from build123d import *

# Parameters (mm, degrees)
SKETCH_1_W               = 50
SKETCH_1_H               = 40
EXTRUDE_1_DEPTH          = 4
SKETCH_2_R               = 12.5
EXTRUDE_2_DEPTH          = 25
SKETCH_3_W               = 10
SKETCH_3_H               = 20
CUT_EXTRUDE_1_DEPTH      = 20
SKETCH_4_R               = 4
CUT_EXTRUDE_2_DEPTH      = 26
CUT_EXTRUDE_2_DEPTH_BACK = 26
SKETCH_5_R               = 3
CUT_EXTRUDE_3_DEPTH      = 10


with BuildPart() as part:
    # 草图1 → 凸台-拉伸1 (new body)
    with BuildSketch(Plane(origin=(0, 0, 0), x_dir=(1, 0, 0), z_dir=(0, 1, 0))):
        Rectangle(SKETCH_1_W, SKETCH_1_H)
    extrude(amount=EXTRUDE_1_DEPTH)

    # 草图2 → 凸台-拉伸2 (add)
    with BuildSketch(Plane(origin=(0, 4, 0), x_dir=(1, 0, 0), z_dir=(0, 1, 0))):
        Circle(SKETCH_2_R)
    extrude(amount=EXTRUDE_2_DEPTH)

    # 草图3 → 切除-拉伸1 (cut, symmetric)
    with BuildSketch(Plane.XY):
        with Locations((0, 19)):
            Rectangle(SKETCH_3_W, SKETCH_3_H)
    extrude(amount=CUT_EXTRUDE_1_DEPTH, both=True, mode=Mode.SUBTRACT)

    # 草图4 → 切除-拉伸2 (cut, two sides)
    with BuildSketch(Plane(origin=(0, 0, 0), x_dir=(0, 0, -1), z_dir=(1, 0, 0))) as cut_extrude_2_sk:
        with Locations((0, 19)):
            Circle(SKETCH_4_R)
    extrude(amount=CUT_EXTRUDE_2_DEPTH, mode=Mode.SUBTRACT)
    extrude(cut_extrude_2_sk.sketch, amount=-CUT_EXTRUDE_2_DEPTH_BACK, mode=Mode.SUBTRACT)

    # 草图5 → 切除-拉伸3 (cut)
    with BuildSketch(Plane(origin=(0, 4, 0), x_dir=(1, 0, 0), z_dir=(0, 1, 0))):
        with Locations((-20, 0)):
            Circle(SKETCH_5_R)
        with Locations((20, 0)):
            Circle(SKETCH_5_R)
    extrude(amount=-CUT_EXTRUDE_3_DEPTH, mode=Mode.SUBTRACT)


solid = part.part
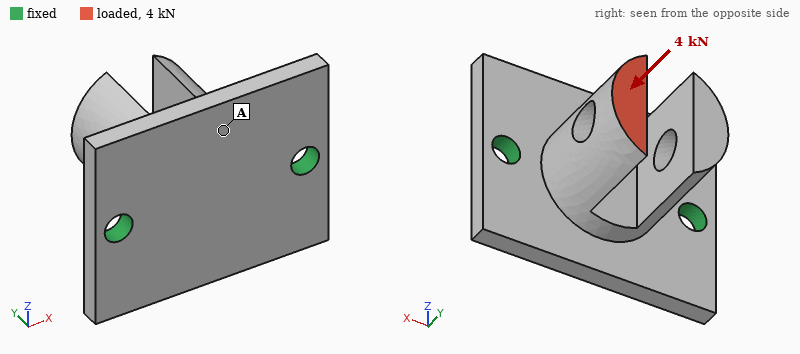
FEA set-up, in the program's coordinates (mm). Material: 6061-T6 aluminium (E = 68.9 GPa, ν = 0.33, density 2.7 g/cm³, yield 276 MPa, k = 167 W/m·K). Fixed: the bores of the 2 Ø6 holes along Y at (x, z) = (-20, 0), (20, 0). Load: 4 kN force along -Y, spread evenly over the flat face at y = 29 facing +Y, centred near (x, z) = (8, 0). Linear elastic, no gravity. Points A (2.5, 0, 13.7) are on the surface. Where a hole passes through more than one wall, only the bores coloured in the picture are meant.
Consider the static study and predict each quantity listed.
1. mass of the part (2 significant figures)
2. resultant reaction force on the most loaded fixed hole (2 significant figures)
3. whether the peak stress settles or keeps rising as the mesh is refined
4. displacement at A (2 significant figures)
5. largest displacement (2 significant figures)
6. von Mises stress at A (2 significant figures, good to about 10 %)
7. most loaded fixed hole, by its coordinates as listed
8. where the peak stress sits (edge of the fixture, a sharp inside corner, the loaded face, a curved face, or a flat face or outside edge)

39 g
3.2 kN
keeps rising
38 µm
64 µm
28 MPa
(20, 0)
edge of the fixture
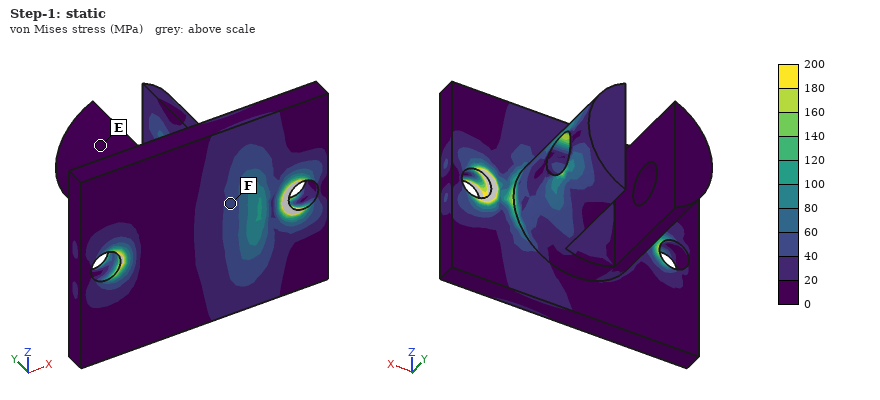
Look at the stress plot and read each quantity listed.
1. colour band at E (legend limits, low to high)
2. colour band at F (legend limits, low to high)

0 to 20 MPa
40 to 60 MPa
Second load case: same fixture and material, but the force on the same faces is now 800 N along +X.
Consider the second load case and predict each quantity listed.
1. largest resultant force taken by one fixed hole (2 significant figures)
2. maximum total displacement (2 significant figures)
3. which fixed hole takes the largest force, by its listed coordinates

1.1 kN
0.18 mm
(-20, 0)
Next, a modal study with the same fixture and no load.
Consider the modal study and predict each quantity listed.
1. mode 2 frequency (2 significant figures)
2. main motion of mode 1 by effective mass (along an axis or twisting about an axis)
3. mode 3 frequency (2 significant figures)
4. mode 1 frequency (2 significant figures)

7900 Hz
along Z
8000 Hz
4000 Hz
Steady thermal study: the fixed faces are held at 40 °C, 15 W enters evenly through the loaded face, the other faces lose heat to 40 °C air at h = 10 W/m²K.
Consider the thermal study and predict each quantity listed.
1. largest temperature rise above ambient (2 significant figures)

28 K
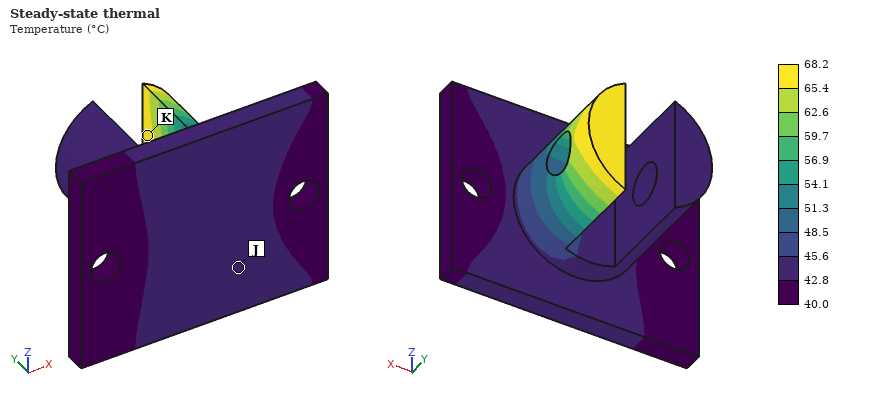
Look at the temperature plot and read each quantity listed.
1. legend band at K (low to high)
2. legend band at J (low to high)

65.4 to 68.2 °C
42.8 to 45.6 °C
